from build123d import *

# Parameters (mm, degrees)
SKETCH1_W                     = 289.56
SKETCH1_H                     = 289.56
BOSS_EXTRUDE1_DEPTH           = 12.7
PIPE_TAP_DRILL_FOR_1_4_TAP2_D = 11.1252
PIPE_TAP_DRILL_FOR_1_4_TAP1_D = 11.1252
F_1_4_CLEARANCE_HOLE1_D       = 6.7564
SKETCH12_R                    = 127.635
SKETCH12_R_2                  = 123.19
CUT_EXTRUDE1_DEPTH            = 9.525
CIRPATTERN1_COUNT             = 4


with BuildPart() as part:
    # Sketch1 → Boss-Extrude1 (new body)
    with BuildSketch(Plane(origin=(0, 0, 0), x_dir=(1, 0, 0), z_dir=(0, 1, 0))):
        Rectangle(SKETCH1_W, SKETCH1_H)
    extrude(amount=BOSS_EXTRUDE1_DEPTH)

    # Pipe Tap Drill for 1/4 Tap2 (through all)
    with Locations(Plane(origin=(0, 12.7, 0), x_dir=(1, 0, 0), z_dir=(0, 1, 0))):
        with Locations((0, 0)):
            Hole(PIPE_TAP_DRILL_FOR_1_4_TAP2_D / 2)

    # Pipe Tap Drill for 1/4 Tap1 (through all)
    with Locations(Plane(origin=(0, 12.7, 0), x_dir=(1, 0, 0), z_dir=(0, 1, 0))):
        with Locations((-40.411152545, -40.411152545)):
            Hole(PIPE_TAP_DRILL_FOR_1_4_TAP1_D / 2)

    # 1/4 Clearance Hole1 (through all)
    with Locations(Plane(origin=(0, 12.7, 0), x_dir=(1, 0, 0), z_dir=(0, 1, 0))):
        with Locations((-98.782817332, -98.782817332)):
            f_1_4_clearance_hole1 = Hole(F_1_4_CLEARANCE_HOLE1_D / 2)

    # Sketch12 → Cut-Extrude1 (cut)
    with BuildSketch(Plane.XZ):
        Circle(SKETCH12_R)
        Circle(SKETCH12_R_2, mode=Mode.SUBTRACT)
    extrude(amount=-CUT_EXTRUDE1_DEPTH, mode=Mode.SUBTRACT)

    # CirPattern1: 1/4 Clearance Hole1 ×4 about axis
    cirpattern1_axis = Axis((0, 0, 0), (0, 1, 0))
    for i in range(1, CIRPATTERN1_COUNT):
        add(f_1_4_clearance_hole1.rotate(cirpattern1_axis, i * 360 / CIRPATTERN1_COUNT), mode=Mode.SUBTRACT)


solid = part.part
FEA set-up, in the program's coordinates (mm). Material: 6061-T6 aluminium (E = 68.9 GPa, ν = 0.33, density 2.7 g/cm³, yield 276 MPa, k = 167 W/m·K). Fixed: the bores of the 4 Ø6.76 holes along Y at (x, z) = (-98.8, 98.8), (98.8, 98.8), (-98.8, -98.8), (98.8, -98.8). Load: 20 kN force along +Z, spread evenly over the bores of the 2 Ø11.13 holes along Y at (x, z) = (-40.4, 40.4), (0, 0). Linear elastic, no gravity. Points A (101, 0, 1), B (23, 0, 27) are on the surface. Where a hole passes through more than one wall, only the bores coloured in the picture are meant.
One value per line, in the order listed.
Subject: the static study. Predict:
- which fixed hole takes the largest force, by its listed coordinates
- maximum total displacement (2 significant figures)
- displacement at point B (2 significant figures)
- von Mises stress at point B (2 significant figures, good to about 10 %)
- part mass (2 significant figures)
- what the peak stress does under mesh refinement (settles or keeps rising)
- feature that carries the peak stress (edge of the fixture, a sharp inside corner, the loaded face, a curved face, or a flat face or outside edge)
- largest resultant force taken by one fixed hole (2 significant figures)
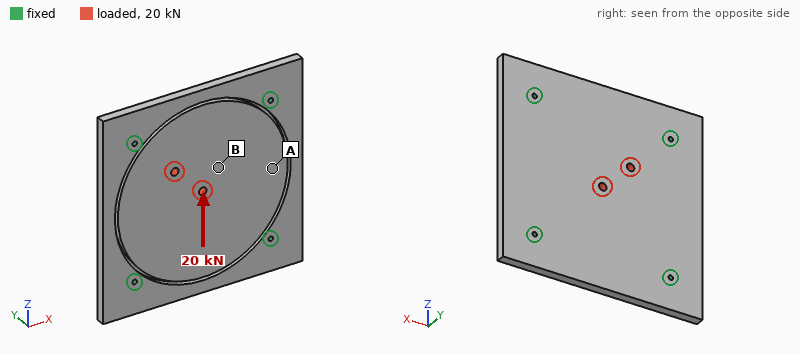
(-98.8, 98.8)
27 µm
18 µm
6.7 MPa
2.8 kg
keeps rising
edge of the fixture
6.2 kN
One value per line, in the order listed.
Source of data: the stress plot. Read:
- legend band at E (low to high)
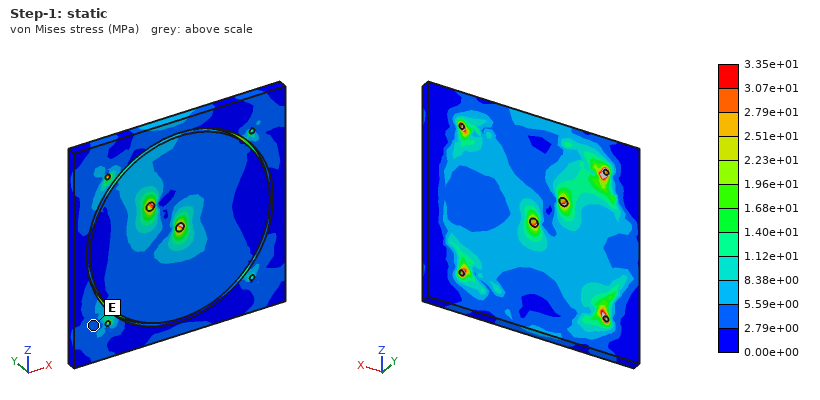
2.79e+00 to 5.59e+00 MPa
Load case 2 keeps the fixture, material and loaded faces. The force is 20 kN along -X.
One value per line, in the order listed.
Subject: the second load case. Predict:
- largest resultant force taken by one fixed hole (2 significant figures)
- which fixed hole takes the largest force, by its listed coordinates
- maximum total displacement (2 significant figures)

6.2 kN
(-98.8, 98.8)
27 µm
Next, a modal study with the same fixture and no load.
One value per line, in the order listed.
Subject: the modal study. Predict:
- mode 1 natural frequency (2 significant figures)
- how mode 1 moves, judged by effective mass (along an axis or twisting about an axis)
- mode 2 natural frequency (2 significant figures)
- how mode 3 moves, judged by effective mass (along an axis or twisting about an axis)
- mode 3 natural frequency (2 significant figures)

920 Hz
along Y
1300 Hz
twisting about X
1400 Hz
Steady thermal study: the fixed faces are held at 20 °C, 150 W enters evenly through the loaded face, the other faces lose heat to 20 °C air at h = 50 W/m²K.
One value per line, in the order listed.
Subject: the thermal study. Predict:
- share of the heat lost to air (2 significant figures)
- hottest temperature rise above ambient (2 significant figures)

48 %
27 K
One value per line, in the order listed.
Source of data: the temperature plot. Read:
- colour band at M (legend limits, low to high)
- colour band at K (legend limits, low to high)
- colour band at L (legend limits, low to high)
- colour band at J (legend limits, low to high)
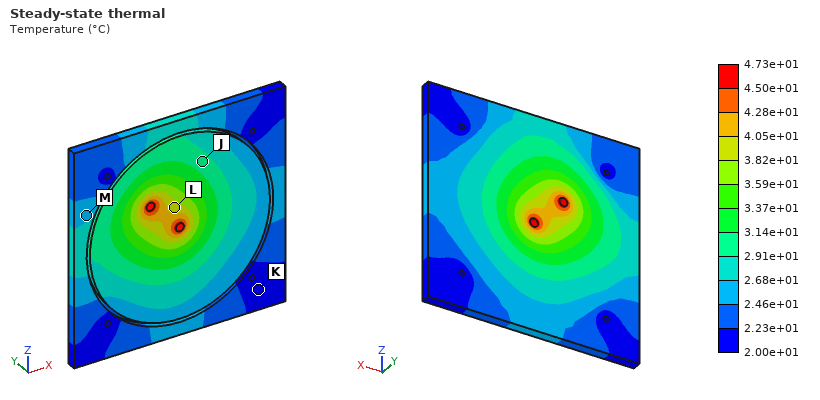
2.46e+01 to 2.68e+01 °C
2.00e+01 to 2.23e+01 °C
3.82e+01 to 4.05e+01 °C
2.91e+01 to 3.14e+01 °C
